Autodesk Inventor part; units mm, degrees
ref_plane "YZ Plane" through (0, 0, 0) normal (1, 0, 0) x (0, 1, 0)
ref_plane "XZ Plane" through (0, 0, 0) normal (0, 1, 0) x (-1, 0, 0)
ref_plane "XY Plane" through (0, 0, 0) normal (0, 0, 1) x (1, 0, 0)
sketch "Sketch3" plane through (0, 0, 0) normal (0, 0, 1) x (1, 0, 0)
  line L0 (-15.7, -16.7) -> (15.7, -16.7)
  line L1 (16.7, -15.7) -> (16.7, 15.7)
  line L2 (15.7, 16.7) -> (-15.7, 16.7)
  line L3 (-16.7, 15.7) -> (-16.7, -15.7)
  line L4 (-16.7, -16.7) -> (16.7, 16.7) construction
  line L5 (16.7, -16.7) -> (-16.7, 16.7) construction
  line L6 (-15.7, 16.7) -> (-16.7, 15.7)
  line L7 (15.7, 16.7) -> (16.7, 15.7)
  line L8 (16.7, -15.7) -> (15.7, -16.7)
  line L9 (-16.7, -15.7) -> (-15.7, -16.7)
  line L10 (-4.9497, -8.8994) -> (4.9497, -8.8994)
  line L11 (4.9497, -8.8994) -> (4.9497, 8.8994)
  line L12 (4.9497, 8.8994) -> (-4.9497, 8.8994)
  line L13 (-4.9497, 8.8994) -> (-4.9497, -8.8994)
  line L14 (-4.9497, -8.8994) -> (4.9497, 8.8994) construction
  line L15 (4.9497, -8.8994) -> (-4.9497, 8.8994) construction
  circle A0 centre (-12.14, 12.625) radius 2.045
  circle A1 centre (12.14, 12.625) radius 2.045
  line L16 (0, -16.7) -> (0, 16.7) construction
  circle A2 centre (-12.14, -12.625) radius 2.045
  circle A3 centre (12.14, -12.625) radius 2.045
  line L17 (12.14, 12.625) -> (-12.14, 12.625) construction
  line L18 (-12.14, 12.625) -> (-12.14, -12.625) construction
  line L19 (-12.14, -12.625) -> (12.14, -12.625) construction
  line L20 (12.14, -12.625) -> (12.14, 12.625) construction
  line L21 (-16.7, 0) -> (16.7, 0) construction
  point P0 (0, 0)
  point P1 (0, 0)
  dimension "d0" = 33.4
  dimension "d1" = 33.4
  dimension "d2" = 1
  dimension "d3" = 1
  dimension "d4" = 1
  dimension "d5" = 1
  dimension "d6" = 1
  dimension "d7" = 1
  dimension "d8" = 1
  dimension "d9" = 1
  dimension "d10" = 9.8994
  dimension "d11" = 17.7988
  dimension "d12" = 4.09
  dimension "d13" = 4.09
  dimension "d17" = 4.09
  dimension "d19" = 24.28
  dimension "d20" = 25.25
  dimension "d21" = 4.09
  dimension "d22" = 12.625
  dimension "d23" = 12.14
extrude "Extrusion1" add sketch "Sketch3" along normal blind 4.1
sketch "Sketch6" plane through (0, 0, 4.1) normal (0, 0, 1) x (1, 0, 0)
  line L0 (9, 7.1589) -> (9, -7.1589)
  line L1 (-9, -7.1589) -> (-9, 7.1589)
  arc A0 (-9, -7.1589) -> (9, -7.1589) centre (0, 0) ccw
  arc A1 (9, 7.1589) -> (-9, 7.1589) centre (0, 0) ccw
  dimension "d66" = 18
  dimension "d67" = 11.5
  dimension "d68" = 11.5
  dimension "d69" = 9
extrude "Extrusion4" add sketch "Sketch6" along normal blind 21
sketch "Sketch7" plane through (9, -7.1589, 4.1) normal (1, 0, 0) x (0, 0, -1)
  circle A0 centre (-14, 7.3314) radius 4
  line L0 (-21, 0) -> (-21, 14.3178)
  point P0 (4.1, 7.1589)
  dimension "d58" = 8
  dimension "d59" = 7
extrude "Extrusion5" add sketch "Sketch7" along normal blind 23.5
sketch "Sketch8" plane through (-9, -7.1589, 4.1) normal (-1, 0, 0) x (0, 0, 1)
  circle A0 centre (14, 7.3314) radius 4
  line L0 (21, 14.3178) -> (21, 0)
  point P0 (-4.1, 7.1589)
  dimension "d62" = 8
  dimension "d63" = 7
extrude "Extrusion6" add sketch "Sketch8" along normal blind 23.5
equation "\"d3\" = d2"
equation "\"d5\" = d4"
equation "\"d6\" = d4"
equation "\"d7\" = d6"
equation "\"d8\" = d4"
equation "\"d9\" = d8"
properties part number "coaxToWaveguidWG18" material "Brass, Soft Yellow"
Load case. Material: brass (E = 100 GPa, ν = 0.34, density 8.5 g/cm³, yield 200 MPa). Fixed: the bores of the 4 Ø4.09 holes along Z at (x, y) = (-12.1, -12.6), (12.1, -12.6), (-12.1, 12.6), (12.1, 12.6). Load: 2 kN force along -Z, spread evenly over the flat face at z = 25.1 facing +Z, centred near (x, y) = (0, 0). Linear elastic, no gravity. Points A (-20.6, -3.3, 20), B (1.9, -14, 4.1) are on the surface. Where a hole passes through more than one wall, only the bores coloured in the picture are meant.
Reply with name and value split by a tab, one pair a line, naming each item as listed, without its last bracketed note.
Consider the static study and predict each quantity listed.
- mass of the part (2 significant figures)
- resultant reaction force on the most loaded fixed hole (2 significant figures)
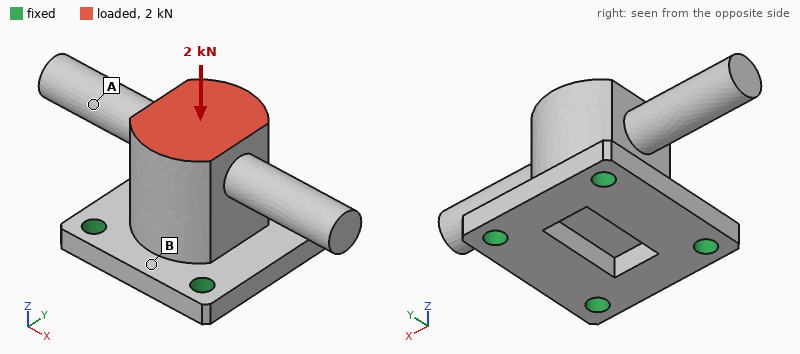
mass of the part	120 g
resultant reaction force on the most loaded fixed hole	570 N
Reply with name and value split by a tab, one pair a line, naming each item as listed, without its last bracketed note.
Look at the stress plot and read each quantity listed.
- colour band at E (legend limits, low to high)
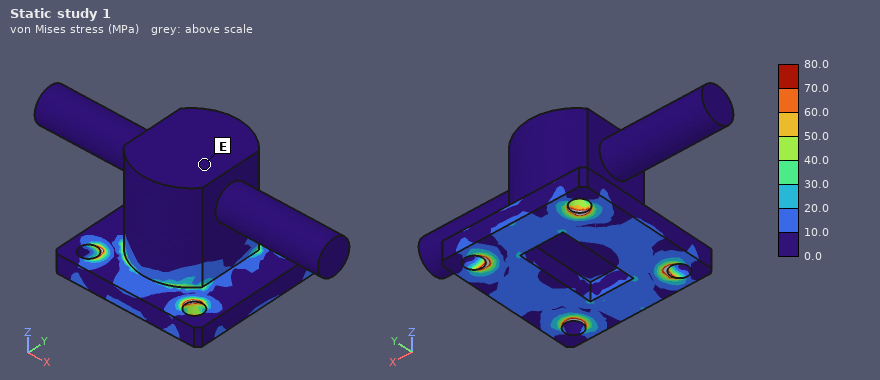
colour band at E	0.0 to 10.0 MPa
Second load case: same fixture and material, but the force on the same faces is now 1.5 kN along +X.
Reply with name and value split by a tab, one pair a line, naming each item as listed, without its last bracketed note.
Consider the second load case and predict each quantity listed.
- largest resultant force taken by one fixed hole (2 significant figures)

largest resultant force taken by one fixed hole	970 N
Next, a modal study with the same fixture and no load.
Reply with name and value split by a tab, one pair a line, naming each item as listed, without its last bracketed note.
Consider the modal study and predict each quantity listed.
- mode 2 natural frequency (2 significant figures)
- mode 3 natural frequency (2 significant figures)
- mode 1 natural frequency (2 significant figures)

mode 2 natural frequency	5100 Hz
mode 3 natural frequency	5100 Hz
mode 1 natural frequency	4100 Hz
